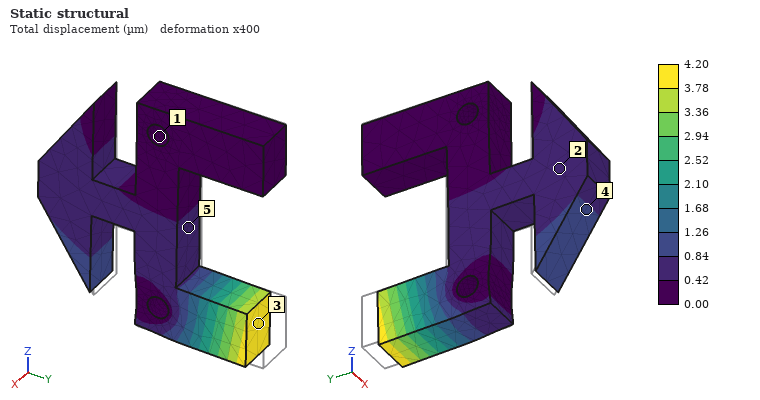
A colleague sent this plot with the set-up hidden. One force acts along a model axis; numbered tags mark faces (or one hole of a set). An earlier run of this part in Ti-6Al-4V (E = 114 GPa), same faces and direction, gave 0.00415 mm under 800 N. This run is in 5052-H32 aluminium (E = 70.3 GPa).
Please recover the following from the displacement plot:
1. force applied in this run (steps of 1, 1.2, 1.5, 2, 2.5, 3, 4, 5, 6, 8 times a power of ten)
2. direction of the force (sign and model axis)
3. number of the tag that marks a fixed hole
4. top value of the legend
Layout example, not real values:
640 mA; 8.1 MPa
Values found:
500 N; -Y; 1; 4.20 µm
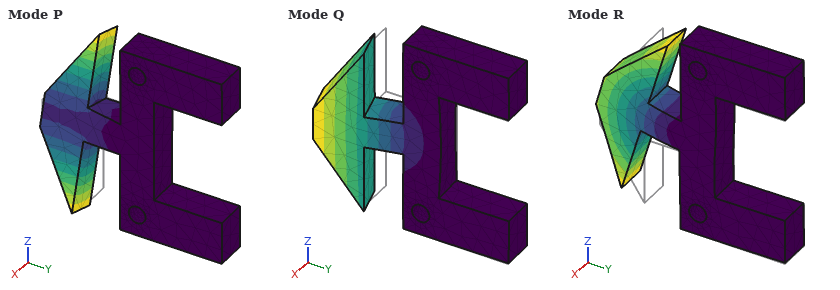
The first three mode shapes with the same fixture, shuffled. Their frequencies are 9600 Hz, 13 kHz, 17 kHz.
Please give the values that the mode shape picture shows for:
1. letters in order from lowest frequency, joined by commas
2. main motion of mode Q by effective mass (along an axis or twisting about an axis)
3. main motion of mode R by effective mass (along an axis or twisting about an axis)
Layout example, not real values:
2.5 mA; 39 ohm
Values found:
Q, R, P; along X; along Z
